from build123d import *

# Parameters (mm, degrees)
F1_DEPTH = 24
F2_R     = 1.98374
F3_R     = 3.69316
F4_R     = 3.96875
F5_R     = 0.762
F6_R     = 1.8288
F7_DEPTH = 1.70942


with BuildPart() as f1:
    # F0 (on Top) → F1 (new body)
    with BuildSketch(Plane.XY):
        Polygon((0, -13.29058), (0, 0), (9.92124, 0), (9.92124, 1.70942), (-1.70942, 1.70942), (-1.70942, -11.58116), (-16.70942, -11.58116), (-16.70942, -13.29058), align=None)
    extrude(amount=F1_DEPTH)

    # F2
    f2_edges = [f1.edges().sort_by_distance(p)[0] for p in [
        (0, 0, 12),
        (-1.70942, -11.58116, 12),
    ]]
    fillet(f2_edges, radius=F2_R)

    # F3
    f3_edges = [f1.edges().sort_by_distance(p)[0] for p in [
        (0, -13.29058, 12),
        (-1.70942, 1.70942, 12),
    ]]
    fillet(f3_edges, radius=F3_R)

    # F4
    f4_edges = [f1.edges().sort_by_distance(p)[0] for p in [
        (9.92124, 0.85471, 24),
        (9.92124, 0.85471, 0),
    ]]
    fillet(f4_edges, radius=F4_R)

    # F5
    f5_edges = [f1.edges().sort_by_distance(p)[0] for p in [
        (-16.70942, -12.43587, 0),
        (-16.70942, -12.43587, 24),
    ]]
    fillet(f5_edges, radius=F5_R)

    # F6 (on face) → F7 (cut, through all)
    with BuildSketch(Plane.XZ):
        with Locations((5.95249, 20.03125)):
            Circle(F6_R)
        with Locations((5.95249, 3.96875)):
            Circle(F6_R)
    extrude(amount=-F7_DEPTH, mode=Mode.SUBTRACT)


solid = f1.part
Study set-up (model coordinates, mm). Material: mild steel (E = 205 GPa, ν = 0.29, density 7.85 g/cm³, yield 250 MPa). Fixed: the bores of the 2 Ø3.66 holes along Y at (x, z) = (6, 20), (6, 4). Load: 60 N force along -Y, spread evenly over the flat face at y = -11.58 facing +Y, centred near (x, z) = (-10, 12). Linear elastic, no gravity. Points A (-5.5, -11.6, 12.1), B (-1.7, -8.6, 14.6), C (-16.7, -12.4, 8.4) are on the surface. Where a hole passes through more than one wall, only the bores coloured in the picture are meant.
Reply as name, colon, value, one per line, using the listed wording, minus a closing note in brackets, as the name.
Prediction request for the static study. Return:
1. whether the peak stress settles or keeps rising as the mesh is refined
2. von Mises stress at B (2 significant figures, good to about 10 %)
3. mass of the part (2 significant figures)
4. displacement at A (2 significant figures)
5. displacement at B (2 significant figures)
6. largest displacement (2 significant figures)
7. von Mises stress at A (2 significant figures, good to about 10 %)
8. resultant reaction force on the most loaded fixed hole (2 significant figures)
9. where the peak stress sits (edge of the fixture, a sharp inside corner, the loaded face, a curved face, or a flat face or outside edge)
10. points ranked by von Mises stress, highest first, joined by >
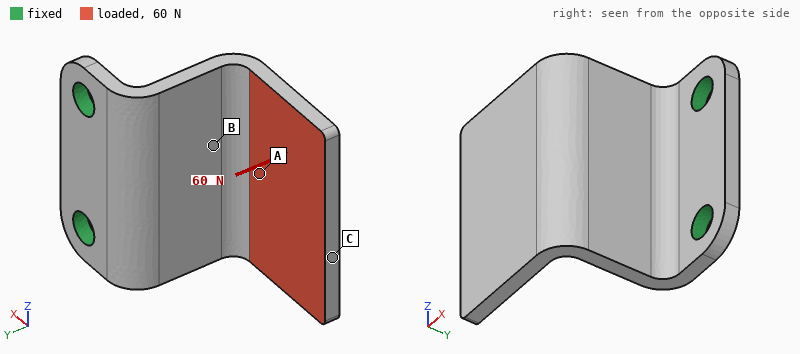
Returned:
whether the peak stress settles or keeps rising as the mesh is refined: keeps rising
von Mises stress at B: 44 MPa
mass of the part: 12 g
displacement at A: 0.052 mm
displacement at B: 0.030 mm
largest displacement: 0.11 mm
von Mises stress at A: 23 MPa
resultant reaction force on the most loaded fixed hole: 30 N
where the peak stress sits: edge of the fixture
points ranked by von Mises stress, highest first, joined by >: B > A > C
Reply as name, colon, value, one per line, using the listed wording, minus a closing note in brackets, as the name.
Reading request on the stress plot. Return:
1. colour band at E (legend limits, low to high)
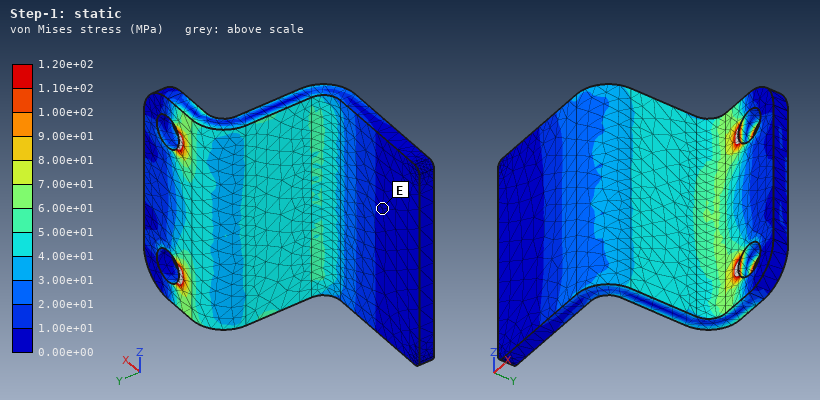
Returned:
colour band at E: 0.00e+00 to 1.00e+01 MPa
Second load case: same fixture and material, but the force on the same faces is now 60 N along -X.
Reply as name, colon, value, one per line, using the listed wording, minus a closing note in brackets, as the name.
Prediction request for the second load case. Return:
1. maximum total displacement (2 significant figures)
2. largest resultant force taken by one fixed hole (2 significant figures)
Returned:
maximum total displacement: 78 µm
largest resultant force taken by one fixed hole: 31 N
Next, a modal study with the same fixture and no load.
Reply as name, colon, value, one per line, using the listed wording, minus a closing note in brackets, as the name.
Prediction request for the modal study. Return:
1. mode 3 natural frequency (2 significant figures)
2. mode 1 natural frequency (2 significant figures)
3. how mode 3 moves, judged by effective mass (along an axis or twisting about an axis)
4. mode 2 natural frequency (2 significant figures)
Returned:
mode 3 natural frequency: 6200 Hz
mode 1 natural frequency: 1700 Hz
how mode 3 moves, judged by effective mass: along X
mode 2 natural frequency: 4000 Hz
